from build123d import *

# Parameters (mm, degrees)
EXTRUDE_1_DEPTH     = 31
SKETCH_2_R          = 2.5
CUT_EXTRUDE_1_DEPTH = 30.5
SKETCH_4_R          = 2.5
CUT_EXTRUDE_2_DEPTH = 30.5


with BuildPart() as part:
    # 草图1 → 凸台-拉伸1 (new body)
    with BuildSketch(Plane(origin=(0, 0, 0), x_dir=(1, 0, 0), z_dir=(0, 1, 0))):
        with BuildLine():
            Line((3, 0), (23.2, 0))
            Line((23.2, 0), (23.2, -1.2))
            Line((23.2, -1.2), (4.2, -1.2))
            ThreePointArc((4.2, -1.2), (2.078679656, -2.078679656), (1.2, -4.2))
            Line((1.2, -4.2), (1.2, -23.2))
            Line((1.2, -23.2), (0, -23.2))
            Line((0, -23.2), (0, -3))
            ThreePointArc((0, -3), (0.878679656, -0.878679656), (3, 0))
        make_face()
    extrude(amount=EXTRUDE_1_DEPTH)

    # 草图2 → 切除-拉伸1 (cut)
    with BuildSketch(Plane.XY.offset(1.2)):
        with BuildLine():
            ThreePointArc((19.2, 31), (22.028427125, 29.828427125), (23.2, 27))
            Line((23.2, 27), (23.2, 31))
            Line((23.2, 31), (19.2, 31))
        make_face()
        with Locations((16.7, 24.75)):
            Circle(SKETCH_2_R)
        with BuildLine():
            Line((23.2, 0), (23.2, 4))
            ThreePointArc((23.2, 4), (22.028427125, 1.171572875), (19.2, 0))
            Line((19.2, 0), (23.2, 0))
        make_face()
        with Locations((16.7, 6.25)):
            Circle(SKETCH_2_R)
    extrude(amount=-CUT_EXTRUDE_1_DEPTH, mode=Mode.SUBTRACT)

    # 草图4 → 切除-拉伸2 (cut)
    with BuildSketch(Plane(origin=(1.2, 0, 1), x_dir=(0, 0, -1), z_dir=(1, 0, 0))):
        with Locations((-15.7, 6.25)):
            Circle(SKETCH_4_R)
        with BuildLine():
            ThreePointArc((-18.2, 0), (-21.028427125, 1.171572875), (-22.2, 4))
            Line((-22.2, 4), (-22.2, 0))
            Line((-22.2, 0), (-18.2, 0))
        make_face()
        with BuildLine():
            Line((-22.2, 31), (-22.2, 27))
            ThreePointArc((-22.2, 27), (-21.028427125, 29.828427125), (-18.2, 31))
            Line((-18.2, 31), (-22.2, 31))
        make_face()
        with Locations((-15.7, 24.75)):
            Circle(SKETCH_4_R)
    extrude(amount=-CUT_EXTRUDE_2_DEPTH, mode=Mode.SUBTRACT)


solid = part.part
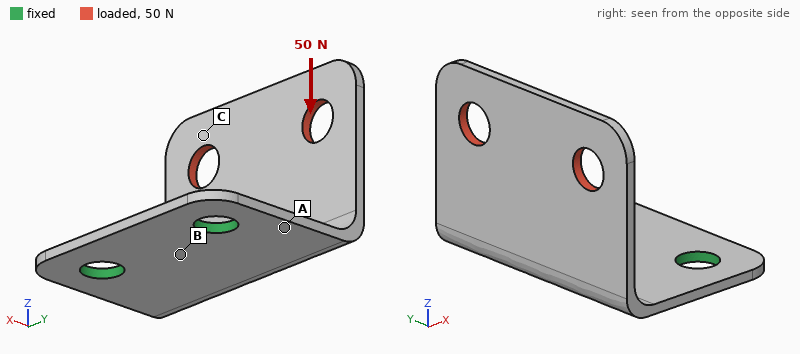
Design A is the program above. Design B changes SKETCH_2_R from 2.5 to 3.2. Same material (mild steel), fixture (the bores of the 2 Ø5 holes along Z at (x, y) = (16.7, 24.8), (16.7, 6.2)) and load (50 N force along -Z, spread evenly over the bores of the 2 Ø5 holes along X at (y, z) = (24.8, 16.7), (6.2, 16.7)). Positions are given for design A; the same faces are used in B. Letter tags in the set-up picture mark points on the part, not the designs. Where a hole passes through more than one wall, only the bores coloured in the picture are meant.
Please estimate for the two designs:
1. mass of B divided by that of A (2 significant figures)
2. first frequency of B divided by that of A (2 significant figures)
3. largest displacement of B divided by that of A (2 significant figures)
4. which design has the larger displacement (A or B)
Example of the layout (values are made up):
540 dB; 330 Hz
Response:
0.98; 1.0; 0.88; A
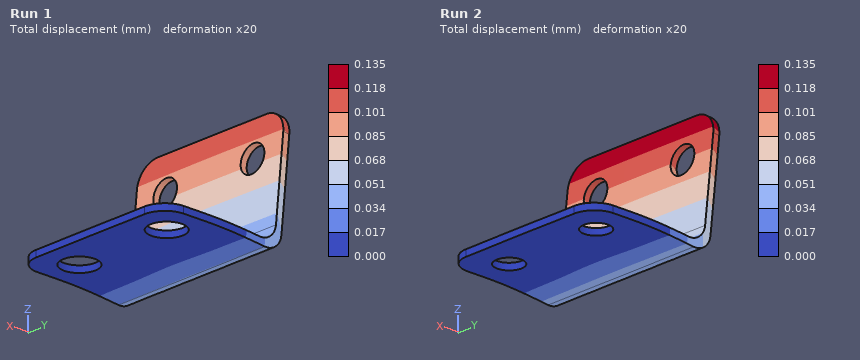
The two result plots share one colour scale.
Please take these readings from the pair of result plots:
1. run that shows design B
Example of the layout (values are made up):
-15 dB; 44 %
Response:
Run 1
